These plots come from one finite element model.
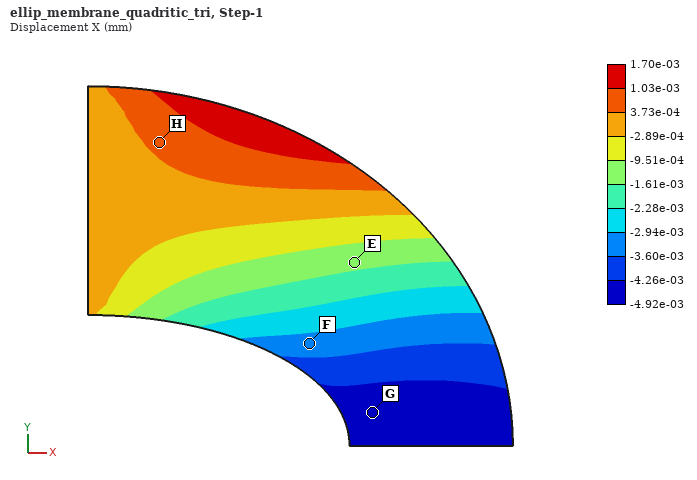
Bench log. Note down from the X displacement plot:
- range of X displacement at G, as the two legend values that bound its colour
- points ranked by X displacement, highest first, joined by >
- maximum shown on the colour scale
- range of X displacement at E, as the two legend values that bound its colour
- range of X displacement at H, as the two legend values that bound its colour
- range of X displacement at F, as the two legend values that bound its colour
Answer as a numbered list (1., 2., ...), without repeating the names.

1. -4.92e-03 to -4.26e-03 mm
2. H > E > F > G
3. 1.70e-03 mm
4. -1.61e-03 to -9.51e-04 mm
5. 3.73e-04 to 1.03e-03 mm
6. -3.60e-03 to -2.94e-03 mm
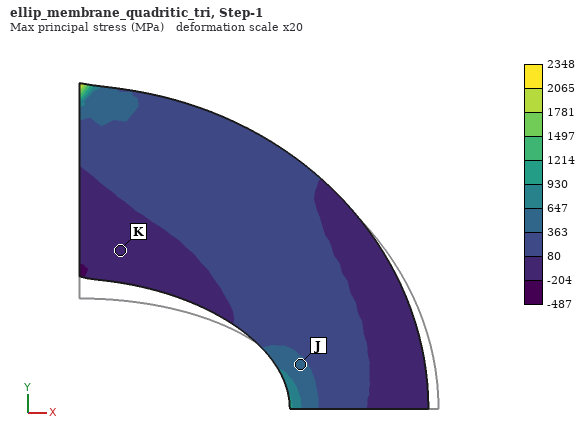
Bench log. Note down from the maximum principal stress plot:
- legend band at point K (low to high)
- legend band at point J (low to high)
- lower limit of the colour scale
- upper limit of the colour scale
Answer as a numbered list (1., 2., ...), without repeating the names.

1. -204 to 80 MPa
2. 363 to 647 MPa
3. -487 MPa
4. 2348 MPa
